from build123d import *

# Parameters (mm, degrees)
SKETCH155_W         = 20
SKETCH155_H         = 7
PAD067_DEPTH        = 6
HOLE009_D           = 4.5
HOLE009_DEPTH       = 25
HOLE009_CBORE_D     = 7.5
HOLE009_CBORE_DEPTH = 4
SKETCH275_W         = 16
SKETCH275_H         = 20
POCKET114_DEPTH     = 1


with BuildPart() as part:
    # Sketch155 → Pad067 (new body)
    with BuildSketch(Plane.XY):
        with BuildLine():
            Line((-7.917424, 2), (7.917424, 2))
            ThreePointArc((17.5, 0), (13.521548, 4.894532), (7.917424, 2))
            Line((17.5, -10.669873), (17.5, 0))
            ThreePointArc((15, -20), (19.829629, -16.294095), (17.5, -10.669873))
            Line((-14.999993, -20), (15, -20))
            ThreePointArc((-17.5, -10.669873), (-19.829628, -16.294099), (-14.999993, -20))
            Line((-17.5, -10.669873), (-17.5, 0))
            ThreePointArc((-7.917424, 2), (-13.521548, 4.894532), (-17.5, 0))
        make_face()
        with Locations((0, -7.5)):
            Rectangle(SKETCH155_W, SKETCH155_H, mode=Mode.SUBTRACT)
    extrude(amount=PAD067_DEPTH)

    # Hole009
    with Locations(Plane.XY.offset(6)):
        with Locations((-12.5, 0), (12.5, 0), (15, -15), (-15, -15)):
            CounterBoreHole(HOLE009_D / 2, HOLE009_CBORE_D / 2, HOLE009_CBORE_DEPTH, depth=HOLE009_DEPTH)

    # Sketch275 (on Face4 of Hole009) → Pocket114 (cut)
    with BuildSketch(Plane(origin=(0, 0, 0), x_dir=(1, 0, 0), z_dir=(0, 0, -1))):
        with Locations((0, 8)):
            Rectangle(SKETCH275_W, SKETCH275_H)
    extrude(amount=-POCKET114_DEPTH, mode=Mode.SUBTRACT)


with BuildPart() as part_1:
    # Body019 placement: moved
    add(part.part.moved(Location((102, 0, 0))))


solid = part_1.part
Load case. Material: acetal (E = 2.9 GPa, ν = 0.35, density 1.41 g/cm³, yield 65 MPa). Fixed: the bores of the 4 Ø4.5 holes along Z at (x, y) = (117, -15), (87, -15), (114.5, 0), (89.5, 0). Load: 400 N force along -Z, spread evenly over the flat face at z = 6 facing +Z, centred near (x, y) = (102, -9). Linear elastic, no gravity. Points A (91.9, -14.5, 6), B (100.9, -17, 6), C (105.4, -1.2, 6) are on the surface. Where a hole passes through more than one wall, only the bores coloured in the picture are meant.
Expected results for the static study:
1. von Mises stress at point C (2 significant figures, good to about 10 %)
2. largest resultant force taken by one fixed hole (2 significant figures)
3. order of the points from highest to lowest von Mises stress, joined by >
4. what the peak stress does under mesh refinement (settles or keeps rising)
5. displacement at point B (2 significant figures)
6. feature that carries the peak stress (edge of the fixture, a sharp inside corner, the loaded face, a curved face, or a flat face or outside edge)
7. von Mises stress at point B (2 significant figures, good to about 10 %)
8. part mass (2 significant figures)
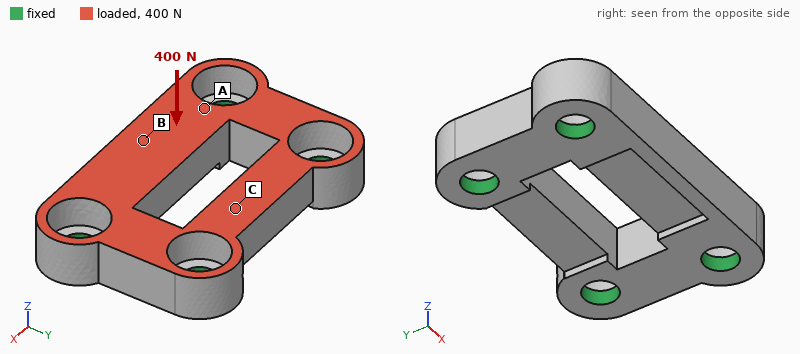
4.0 MPa
150 N
B > C > A
keeps rising
65 µm
edge of the fixture
7.1 MPa
4.4 g
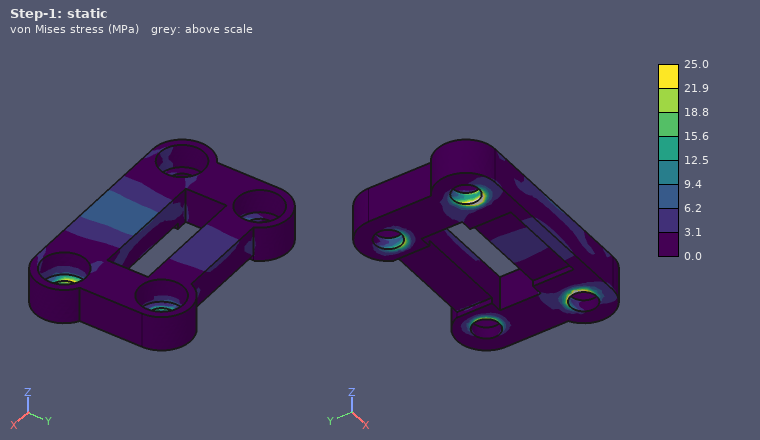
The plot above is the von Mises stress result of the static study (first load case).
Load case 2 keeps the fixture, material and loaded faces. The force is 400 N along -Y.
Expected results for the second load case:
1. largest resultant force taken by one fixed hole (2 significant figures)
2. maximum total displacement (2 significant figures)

120 N
72 µm
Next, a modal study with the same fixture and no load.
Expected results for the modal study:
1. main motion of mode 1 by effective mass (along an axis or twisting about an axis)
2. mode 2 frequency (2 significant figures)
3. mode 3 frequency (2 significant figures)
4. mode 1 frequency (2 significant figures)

along Z
9600 Hz
9900 Hz
6900 Hz
